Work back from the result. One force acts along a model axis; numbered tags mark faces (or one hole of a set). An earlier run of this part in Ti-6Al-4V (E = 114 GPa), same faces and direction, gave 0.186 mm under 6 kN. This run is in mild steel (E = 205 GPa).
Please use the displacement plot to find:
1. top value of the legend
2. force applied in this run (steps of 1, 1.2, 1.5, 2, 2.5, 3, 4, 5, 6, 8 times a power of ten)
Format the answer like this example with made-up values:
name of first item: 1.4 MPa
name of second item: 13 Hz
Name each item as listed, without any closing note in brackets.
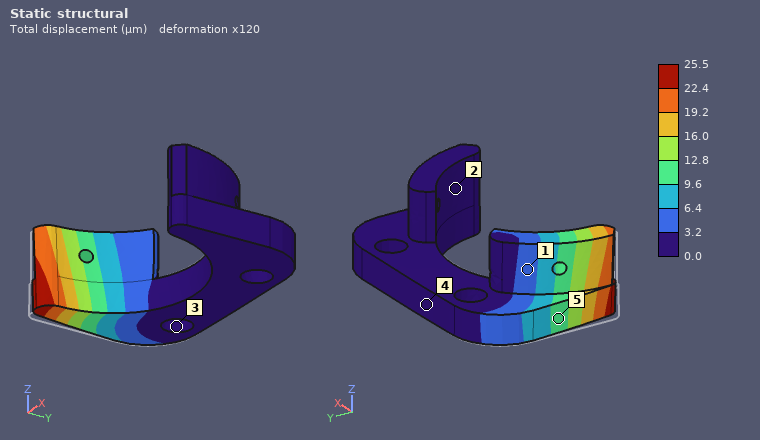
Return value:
top value of the legend: 25.5 µm
force applied in this run: 1.5 kN
